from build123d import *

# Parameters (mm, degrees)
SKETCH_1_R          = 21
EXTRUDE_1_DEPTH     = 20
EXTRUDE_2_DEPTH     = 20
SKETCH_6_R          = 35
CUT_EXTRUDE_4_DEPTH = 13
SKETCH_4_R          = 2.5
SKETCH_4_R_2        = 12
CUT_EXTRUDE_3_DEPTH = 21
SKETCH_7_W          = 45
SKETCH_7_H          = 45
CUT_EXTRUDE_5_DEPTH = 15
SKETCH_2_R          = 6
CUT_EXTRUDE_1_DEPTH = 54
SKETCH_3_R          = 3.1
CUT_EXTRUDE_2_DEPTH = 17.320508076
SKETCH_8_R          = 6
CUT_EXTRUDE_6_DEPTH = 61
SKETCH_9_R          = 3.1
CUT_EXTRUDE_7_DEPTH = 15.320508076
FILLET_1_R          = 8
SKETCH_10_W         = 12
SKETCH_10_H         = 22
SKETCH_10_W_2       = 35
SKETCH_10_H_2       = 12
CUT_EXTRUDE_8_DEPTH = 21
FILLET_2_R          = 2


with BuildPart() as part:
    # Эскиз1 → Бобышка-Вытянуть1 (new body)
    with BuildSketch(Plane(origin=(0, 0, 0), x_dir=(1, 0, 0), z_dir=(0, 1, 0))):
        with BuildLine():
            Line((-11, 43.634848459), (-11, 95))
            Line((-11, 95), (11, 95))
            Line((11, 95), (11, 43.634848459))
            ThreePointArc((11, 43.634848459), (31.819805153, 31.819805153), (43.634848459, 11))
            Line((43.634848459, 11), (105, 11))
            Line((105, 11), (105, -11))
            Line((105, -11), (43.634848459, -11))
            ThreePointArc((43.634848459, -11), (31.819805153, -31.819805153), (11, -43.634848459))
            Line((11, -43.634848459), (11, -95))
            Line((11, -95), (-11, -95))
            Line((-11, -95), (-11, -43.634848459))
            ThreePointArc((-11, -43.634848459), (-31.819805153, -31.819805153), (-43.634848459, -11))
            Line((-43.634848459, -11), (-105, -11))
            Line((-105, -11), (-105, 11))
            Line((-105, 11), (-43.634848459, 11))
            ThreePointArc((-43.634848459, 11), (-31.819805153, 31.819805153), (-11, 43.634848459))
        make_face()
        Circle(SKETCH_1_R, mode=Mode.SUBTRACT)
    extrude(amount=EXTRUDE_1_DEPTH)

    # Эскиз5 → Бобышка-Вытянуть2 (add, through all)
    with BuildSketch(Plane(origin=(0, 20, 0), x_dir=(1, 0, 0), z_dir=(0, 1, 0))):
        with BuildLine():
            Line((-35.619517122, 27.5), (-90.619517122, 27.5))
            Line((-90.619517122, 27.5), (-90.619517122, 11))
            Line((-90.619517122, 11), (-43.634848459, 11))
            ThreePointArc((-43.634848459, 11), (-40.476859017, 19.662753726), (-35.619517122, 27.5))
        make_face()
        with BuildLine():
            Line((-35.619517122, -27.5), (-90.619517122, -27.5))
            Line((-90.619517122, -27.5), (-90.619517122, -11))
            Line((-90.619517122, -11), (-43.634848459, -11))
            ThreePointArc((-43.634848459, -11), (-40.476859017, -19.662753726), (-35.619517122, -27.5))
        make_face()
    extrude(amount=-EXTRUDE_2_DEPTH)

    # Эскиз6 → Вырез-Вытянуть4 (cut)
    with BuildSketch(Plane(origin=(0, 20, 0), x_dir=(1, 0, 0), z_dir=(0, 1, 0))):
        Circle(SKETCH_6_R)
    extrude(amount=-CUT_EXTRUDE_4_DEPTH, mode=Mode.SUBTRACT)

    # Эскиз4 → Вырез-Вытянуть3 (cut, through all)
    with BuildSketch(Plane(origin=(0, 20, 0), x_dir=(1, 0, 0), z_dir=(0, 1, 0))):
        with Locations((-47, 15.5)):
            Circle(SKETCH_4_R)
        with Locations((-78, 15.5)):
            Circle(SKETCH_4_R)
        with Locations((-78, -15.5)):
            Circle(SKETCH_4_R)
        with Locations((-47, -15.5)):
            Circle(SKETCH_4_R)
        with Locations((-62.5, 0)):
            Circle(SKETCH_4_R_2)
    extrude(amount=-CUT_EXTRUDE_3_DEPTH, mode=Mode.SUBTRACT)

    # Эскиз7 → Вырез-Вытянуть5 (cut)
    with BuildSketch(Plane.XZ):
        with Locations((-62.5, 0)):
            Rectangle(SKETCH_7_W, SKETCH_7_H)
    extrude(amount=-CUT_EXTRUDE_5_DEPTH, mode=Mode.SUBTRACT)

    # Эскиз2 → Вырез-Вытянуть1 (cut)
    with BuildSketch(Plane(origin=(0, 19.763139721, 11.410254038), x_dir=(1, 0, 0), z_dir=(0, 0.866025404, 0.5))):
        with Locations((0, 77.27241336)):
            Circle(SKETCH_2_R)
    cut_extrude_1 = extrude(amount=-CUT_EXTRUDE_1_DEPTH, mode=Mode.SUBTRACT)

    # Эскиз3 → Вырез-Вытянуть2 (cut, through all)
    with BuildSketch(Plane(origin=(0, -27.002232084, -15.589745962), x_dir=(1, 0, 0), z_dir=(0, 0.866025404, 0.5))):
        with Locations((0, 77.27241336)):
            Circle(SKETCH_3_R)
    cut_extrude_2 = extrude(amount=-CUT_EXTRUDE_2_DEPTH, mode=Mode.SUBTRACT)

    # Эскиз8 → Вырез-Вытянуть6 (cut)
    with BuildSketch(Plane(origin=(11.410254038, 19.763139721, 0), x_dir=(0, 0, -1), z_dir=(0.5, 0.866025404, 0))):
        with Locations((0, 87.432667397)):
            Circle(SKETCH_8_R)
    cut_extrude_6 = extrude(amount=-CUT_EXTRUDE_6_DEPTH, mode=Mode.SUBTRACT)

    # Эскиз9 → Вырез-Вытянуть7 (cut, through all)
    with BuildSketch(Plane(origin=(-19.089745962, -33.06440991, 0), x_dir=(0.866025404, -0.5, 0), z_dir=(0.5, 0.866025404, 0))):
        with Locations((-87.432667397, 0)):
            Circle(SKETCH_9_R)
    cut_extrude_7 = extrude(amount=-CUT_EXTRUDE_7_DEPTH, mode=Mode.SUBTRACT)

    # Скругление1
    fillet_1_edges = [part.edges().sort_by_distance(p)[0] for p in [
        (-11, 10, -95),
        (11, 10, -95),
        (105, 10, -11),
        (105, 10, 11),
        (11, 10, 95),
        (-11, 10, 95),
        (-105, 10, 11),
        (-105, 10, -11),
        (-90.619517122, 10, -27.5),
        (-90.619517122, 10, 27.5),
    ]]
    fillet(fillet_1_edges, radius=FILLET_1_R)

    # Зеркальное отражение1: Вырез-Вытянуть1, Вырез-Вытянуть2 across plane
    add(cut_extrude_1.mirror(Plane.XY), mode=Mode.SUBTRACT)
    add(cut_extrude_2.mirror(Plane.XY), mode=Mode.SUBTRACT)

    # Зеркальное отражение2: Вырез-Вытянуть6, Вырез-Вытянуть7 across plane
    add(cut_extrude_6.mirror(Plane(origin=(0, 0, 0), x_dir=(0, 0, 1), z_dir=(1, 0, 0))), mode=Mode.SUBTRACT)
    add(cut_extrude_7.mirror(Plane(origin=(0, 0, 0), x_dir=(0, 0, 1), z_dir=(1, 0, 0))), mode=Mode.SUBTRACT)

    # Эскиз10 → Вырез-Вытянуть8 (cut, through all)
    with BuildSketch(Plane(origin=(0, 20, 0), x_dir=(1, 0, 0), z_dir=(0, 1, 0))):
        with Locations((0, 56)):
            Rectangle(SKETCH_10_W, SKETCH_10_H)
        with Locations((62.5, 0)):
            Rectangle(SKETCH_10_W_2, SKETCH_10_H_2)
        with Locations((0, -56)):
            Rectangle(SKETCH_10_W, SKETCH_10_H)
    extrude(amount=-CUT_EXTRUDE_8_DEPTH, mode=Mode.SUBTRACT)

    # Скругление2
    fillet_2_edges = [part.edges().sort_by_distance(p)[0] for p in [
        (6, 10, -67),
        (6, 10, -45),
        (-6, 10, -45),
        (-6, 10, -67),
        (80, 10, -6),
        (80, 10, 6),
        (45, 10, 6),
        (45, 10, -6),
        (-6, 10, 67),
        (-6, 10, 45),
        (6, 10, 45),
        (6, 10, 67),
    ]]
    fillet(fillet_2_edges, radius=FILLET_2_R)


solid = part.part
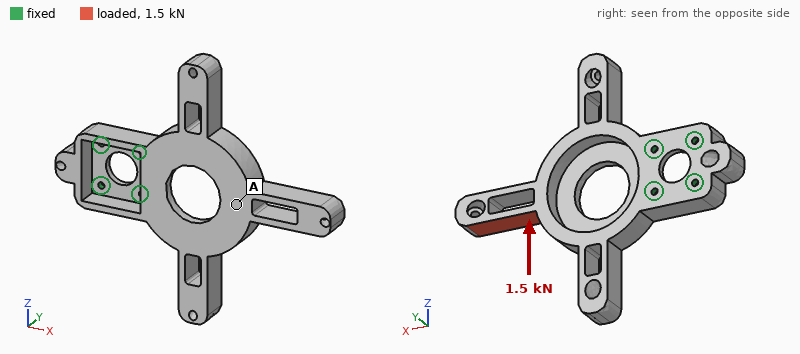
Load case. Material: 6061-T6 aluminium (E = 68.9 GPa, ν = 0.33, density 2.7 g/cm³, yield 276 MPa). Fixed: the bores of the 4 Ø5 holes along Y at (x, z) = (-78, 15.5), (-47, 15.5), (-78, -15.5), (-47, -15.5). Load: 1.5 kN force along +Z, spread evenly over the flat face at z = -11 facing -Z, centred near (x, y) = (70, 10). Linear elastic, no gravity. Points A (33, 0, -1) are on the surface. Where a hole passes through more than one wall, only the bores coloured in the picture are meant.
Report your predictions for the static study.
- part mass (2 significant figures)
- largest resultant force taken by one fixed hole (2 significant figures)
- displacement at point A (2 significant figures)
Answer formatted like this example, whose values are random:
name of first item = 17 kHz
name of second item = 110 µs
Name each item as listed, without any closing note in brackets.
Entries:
part mass = 370 g
largest resultant force taken by one fixed hole = 2.7 kN
displacement at point A = 0.12 mm
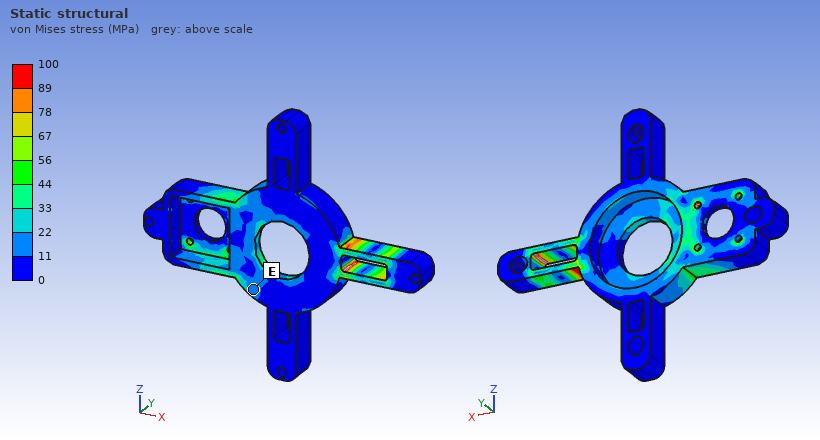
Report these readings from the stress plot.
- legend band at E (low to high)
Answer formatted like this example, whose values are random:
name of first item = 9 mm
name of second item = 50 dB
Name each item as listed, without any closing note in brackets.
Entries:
legend band at E = 11 to 22 MPa
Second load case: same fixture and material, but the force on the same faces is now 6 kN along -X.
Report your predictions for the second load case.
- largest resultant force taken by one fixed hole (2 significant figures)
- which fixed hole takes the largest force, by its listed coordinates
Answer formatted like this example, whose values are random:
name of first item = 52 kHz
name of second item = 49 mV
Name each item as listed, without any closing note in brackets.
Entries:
largest resultant force taken by one fixed hole = 2.8 kN
which fixed hole takes the largest force, by its listed coordinates = (-47, -15.5)
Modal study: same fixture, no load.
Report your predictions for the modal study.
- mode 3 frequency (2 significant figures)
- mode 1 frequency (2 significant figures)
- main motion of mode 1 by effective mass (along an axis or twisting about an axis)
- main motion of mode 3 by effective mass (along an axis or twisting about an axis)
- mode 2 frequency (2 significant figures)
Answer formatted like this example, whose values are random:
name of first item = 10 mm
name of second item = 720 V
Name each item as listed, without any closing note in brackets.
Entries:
mode 3 frequency = 1300 Hz
mode 1 frequency = 540 Hz
main motion of mode 1 by effective mass = along Y
main motion of mode 3 by effective mass = along Z
mode 2 frequency = 850 Hz
